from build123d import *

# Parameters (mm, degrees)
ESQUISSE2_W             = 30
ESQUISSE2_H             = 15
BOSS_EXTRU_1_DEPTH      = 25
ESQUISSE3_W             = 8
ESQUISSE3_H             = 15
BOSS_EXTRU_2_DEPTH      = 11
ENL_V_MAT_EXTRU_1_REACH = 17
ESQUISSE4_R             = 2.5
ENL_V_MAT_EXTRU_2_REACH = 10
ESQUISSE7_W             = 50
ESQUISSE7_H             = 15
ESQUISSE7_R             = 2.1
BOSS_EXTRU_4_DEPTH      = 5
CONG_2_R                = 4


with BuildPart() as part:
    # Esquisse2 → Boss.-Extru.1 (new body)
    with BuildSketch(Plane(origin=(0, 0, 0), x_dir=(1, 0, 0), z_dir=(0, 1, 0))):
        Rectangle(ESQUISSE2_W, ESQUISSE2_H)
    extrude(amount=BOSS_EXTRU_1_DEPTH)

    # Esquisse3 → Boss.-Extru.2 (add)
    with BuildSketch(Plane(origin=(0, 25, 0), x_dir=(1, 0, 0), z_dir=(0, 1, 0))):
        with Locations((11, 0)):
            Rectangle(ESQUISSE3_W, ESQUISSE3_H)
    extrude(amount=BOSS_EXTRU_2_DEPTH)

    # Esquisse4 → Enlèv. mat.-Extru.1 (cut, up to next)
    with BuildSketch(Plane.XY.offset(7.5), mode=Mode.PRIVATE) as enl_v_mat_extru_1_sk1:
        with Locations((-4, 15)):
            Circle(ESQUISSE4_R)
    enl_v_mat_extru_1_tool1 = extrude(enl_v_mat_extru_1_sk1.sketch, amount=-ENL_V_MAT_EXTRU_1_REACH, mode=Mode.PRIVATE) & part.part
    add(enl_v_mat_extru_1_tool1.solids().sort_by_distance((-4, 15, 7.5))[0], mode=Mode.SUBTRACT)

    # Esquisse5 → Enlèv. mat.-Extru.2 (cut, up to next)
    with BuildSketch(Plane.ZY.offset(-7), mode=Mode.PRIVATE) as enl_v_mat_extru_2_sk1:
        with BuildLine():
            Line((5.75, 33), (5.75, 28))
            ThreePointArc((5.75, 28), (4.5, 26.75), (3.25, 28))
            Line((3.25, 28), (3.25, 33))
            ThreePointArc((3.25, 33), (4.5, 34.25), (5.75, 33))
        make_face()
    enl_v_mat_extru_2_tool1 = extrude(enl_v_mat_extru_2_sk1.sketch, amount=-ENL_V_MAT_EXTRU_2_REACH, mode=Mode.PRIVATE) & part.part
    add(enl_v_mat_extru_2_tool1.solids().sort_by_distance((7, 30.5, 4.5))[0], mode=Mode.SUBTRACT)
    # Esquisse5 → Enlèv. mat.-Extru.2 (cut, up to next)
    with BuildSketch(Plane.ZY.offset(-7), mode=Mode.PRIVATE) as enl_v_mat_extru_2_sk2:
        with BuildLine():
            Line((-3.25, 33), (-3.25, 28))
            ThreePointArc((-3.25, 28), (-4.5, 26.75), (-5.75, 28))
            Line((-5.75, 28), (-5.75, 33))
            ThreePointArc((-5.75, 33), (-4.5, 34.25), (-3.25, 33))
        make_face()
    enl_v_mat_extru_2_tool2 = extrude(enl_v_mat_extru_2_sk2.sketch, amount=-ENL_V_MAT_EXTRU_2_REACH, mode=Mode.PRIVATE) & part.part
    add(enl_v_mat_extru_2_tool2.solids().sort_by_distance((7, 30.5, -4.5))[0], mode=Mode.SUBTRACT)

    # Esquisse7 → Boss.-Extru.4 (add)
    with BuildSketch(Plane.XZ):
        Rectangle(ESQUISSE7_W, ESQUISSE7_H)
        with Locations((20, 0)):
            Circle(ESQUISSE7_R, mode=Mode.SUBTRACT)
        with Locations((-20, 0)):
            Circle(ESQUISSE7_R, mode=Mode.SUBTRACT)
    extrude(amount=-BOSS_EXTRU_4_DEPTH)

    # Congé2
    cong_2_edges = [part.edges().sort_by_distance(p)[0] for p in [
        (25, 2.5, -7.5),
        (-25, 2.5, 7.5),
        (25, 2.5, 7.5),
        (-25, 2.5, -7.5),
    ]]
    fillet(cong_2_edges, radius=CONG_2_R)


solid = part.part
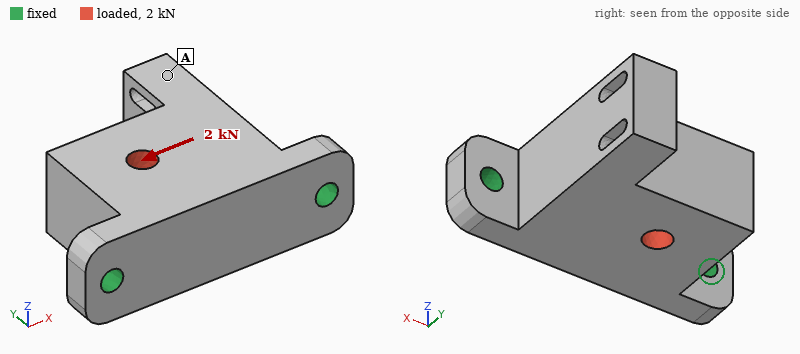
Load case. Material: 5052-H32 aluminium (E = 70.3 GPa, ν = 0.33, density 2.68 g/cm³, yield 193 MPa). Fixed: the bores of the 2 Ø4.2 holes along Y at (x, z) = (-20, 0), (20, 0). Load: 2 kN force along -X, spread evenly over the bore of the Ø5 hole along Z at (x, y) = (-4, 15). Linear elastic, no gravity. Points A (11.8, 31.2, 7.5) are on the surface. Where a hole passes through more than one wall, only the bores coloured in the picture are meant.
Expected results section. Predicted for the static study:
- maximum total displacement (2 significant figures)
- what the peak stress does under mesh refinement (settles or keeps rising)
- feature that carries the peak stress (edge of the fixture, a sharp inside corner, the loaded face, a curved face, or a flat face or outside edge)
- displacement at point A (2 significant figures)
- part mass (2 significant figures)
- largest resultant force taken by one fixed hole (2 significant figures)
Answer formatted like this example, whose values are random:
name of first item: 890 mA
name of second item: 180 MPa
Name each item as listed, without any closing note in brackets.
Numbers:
maximum total displacement: 14 µm
what the peak stress does under mesh refinement: keeps rising
feature that carries the peak stress: edge of the fixture
displacement at point A: 13 µm
part mass: 36 g
largest resultant force taken by one fixed hole: 1.2 kN
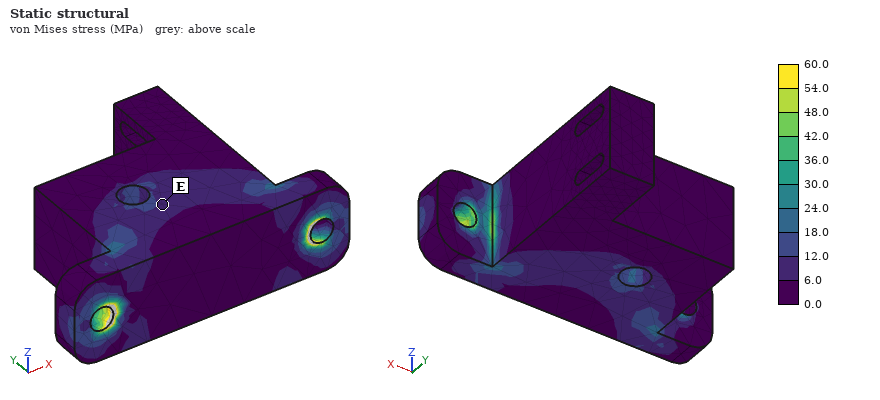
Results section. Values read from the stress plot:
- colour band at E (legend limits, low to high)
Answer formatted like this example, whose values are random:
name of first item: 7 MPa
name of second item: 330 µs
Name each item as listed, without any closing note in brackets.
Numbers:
colour band at E: 6.0 to 12.0 MPa
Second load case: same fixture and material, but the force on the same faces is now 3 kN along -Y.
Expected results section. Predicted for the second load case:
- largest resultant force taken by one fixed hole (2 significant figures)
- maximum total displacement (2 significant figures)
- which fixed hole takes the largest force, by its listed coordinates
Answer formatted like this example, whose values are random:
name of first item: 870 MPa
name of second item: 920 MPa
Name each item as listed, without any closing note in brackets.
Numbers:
largest resultant force taken by one fixed hole: 2.0 kN
maximum total displacement: 15 µm
which fixed hole takes the largest force, by its listed coordinates: (-20, 0)
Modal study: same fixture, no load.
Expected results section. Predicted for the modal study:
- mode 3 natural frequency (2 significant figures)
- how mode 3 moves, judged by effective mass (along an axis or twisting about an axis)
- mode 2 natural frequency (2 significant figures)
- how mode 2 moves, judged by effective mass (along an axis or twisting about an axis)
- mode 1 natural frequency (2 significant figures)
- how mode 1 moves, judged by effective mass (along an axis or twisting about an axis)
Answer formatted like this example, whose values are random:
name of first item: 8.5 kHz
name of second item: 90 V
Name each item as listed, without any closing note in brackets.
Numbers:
mode 3 natural frequency: 14 kHz
how mode 3 moves, judged by effective mass: along Y
mode 2 natural frequency: 13 kHz
how mode 2 moves, judged by effective mass: along X
mode 1 natural frequency: 4100 Hz
how mode 1 moves, judged by effective mass: along Z
